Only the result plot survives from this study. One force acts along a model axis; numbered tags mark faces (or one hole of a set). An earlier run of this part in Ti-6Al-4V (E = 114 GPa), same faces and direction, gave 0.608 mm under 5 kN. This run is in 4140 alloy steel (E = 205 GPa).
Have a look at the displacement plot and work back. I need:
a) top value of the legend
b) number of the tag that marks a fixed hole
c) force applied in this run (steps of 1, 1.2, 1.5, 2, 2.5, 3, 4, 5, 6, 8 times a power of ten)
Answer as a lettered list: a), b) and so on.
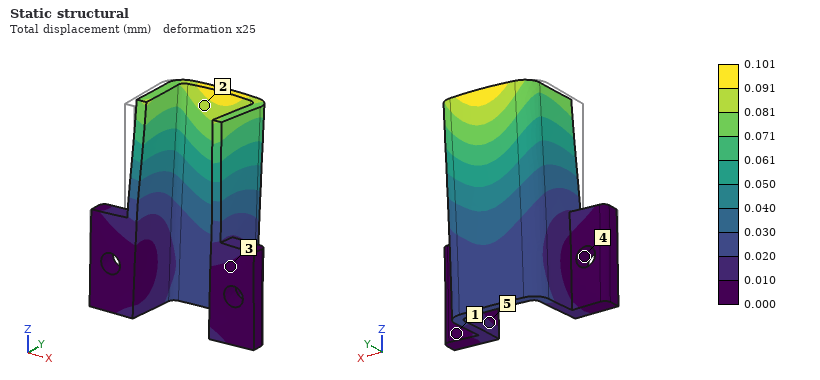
a) 0.101 mm
b) 4
c) 1.5 kN
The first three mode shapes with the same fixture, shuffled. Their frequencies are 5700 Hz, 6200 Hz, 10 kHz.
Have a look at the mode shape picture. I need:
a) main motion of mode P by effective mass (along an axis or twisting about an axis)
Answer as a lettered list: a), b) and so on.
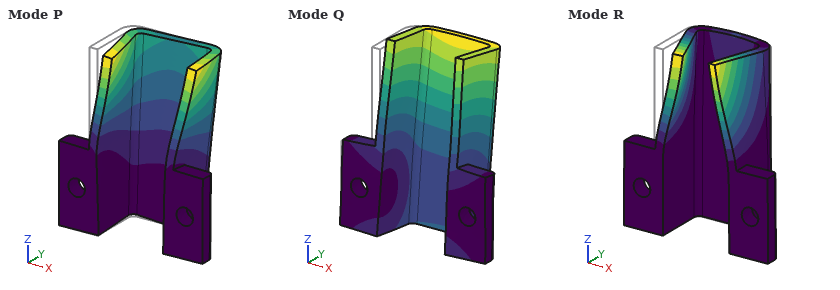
a) along X
